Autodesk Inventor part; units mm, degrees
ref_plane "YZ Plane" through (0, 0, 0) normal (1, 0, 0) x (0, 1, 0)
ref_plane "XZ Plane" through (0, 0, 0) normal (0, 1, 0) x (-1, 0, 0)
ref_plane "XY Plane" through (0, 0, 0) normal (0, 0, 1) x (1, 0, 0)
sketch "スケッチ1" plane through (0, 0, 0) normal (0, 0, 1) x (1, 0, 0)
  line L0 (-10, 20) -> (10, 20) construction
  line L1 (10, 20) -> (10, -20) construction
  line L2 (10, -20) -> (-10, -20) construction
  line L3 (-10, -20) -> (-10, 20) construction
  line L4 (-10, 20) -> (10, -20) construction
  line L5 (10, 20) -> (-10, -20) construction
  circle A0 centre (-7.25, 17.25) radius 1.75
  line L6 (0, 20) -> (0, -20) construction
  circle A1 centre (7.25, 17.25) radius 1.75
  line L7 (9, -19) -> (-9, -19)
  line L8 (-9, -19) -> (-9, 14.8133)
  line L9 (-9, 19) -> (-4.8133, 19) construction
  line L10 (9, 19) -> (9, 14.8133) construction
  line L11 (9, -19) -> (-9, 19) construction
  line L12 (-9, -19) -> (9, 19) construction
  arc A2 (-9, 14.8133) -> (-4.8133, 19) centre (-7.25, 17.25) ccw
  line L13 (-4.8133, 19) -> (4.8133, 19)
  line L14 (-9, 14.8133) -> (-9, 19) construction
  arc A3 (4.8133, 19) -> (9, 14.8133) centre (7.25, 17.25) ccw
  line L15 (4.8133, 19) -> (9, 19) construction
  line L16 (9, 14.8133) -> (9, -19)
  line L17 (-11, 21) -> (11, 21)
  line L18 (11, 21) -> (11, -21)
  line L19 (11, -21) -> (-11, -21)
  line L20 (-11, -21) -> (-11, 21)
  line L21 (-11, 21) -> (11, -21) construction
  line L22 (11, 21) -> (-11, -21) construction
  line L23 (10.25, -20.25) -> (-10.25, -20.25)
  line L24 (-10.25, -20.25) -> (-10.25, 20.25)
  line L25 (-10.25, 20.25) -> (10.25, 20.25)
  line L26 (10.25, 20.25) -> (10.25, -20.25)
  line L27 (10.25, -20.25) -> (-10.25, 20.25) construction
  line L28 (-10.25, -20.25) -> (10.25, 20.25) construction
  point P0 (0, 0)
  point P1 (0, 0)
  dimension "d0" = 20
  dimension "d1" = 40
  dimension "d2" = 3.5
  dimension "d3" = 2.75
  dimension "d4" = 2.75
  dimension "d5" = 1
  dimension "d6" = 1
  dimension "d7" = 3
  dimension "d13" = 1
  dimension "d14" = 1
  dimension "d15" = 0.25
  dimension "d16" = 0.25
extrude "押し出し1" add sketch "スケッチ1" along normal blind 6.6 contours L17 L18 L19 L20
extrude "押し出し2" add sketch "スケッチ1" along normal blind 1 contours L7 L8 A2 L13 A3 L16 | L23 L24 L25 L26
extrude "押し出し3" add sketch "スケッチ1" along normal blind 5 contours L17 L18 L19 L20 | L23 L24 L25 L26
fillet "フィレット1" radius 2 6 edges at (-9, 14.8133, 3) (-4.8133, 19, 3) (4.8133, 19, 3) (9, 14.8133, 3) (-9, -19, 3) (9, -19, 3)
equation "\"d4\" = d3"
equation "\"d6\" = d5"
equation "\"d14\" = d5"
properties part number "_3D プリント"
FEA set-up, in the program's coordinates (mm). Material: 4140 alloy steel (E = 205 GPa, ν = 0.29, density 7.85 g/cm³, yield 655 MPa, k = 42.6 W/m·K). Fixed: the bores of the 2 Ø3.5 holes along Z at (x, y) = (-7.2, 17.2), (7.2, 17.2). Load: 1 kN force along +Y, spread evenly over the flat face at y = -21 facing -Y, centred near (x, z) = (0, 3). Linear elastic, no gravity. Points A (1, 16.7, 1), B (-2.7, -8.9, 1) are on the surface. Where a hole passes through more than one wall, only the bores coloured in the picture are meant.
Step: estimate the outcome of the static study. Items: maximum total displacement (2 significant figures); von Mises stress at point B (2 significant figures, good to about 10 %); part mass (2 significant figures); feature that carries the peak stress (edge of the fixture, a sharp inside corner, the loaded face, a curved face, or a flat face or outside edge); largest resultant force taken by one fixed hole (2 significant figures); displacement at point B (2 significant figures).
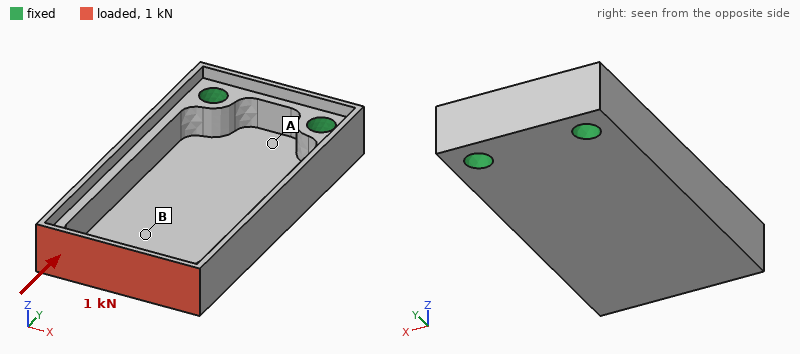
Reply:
68 µm
26 MPa
17 g
a curved face
500 N
22 µm
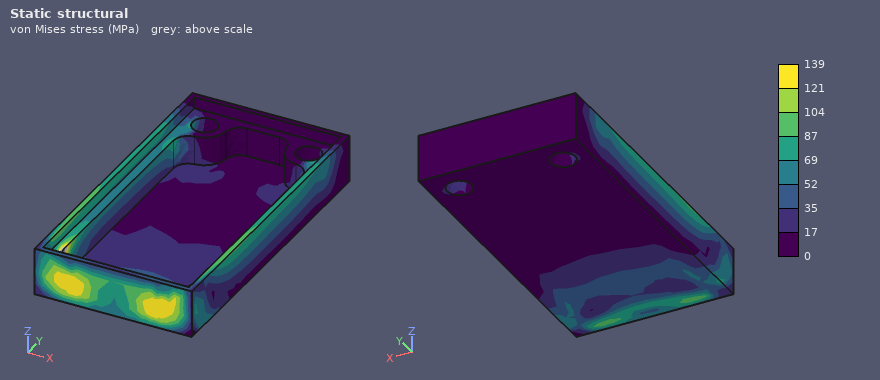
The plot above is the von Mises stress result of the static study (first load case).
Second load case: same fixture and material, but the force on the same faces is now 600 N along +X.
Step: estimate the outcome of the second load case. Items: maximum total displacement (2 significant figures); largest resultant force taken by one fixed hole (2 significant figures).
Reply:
0.19 mm
1.3 kN
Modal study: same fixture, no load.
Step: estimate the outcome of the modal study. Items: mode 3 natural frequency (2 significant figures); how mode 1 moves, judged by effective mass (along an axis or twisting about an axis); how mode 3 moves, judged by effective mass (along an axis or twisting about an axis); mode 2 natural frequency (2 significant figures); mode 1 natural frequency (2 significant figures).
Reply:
10 kHz
along Z
along X
3900 Hz
2700 Hz
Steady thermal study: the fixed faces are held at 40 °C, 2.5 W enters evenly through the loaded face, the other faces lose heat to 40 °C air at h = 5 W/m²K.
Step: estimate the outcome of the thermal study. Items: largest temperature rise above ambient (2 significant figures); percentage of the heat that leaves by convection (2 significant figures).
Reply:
52 K
13 %
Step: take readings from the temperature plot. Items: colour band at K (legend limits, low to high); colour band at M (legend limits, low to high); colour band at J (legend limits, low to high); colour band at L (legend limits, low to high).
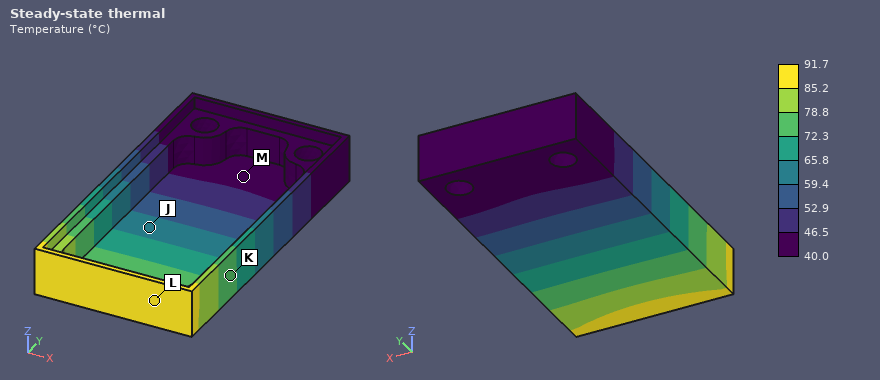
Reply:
72.3 to 78.8 °C
40.0 to 46.5 °C
59.4 to 65.8 °C
85.2 to 91.7 °C
